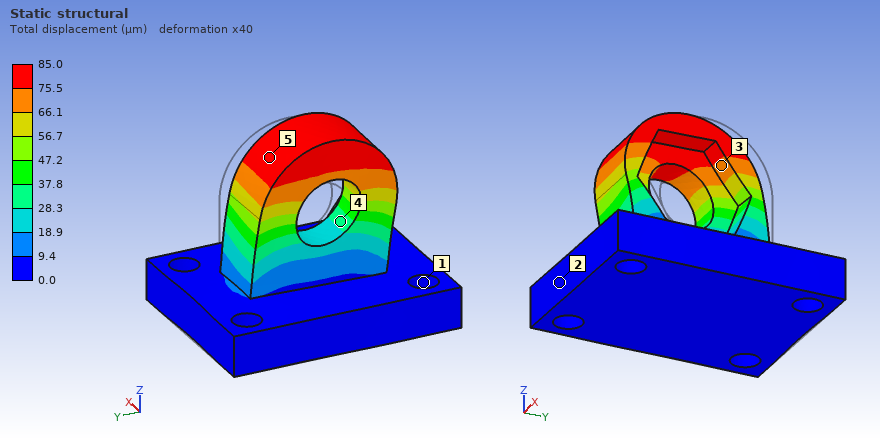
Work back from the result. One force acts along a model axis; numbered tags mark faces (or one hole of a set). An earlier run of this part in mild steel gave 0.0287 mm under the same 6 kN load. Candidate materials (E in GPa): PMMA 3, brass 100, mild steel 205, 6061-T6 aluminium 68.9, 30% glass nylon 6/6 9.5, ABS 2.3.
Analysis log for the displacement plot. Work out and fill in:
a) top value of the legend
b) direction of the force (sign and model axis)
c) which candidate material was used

85.0 µm
-Y
6061-T6 aluminium
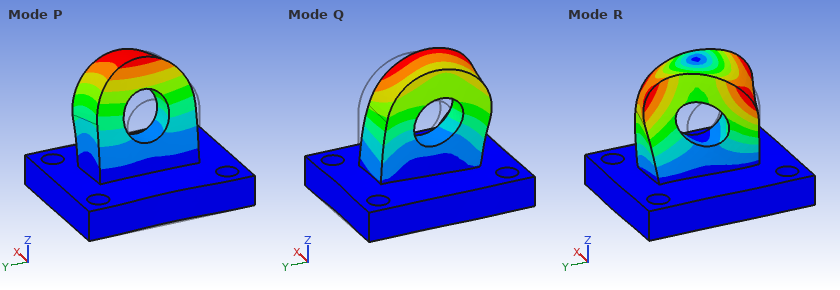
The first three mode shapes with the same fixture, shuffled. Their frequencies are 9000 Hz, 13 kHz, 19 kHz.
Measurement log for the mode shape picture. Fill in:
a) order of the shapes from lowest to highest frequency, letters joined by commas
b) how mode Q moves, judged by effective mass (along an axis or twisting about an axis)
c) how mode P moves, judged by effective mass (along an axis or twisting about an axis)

P, Q, R
along Y
along X
